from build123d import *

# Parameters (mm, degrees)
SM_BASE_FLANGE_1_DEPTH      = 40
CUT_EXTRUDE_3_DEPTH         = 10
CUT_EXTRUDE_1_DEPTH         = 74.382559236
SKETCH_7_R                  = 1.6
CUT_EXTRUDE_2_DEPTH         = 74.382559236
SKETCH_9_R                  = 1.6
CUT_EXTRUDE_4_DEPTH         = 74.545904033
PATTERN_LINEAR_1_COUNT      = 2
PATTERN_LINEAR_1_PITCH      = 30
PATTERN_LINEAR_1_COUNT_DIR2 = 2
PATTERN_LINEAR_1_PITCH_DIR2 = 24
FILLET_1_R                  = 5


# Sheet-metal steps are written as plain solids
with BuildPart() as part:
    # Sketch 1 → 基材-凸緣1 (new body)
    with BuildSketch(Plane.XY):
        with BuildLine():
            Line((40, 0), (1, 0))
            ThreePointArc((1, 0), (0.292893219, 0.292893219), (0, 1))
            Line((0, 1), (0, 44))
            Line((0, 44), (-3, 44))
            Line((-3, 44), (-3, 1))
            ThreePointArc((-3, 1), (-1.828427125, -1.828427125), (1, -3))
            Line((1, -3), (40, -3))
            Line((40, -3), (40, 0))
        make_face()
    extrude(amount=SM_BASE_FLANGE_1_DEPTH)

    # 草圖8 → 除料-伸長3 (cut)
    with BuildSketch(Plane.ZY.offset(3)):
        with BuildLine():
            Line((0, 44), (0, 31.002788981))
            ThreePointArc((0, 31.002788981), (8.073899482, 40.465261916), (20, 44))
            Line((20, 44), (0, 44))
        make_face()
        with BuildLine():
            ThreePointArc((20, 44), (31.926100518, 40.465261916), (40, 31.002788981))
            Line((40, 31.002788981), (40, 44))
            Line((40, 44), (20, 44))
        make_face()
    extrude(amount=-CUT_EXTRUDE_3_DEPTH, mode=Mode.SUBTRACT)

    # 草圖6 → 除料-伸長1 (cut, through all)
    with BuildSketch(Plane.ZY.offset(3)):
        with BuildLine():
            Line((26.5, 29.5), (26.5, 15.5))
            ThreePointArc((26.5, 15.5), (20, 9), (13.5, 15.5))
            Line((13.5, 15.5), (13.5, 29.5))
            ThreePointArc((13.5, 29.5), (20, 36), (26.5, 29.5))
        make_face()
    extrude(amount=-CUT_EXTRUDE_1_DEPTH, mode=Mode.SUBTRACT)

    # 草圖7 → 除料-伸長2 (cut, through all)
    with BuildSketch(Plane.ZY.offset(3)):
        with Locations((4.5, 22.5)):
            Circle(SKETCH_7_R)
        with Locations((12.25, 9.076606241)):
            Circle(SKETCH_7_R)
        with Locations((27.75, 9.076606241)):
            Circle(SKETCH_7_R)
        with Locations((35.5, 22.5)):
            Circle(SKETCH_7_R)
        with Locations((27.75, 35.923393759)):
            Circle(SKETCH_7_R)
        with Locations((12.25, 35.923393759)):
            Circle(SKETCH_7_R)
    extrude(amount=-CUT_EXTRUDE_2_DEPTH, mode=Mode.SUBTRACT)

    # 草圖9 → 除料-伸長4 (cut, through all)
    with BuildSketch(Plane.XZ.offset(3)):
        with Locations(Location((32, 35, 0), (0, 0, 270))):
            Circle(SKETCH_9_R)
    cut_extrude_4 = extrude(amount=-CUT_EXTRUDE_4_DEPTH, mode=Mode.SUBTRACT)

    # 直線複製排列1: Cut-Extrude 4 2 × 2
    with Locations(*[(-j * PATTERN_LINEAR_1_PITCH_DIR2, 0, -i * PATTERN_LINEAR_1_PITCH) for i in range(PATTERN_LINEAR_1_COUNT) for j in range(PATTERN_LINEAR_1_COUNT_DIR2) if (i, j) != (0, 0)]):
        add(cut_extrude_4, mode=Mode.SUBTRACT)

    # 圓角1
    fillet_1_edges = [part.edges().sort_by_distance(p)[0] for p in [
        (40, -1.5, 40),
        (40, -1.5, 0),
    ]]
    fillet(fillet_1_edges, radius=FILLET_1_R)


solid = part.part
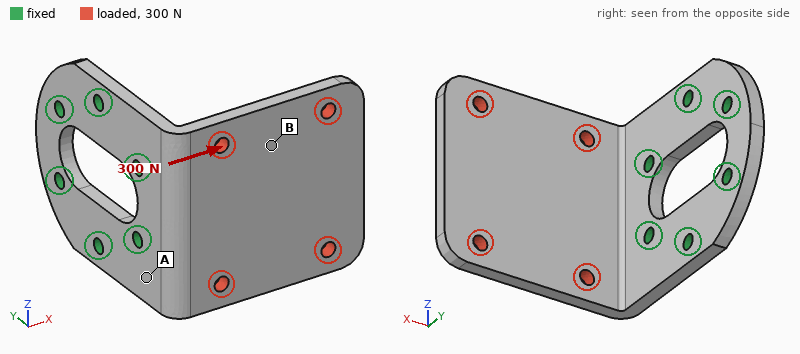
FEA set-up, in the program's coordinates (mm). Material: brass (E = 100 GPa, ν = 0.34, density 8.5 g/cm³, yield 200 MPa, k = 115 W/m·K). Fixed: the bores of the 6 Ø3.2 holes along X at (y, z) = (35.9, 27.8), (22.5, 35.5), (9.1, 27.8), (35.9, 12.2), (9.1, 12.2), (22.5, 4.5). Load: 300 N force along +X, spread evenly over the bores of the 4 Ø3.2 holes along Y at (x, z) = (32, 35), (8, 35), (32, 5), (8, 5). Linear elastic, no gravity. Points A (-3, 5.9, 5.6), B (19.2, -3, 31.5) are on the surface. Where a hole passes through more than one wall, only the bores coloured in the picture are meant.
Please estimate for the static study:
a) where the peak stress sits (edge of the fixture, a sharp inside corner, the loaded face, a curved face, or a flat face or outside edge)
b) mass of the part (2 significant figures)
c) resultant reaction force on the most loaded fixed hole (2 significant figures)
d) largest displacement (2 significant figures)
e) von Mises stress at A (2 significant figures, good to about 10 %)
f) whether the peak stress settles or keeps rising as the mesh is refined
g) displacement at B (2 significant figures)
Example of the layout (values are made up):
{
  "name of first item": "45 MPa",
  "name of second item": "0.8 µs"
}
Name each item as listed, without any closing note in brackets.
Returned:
{
  "where the peak stress sits": "edge of the fixture",
  "mass of the part": "74 g",
  "resultant reaction force on the most loaded fixed hole": "180 N",
  "largest displacement": "85 µm",
  "von Mises stress at A": "25 MPa",
  "whether the peak stress settles or keeps rising as the mesh is refined": "keeps rising",
  "displacement at B": "45 µm"
}
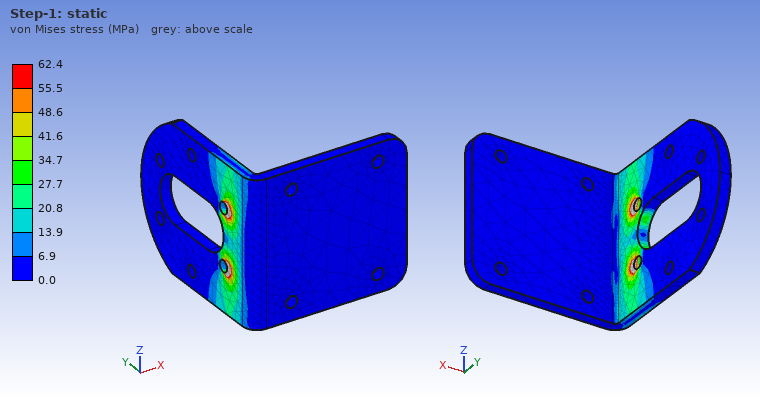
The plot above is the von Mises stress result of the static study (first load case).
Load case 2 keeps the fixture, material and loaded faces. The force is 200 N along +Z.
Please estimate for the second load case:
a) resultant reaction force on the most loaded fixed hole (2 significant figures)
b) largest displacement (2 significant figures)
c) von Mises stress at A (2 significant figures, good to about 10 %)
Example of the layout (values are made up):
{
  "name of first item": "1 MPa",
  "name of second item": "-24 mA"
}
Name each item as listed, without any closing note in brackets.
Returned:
{
  "resultant reaction force on the most loaded fixed hole": "240 N",
  "largest displacement": "56 µm",
  "von Mises stress at A": "19 MPa"
}
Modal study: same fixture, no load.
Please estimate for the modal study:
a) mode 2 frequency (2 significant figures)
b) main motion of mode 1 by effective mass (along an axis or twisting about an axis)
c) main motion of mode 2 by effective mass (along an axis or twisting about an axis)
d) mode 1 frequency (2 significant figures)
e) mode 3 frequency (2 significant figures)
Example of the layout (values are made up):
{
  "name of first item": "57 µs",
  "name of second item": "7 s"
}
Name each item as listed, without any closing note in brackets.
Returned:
{
  "mode 2 frequency": "1700 Hz",
  "main motion of mode 1 by effective mass": "along Y",
  "main motion of mode 2 by effective mass": "along Z",
  "mode 1 frequency": "710 Hz",
  "mode 3 frequency": "2500 Hz"
}
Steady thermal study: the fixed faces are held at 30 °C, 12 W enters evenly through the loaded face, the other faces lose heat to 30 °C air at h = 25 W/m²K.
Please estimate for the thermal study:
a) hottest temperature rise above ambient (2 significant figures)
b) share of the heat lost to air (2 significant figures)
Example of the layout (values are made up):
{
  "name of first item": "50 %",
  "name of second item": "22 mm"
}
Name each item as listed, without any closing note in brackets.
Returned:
{
  "hottest temperature rise above ambient": "27 K",
  "share of the heat lost to air": "15 %"
}
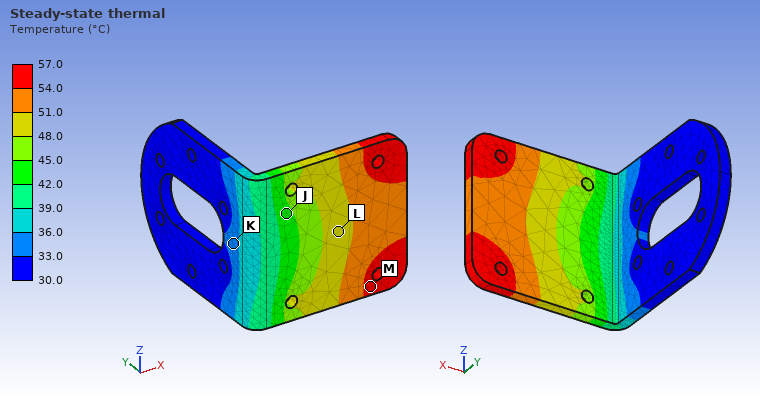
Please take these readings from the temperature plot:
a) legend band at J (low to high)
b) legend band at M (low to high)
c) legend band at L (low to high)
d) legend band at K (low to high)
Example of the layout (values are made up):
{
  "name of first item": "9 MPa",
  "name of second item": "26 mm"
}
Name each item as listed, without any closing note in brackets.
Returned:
{
  "legend band at J": "42.0 to 45.0 °C",
  "legend band at M": "54.0 to 57.0 °C",
  "legend band at L": "48.0 to 51.0 °C",
  "legend band at K": "33.0 to 36.0 °C"
}
